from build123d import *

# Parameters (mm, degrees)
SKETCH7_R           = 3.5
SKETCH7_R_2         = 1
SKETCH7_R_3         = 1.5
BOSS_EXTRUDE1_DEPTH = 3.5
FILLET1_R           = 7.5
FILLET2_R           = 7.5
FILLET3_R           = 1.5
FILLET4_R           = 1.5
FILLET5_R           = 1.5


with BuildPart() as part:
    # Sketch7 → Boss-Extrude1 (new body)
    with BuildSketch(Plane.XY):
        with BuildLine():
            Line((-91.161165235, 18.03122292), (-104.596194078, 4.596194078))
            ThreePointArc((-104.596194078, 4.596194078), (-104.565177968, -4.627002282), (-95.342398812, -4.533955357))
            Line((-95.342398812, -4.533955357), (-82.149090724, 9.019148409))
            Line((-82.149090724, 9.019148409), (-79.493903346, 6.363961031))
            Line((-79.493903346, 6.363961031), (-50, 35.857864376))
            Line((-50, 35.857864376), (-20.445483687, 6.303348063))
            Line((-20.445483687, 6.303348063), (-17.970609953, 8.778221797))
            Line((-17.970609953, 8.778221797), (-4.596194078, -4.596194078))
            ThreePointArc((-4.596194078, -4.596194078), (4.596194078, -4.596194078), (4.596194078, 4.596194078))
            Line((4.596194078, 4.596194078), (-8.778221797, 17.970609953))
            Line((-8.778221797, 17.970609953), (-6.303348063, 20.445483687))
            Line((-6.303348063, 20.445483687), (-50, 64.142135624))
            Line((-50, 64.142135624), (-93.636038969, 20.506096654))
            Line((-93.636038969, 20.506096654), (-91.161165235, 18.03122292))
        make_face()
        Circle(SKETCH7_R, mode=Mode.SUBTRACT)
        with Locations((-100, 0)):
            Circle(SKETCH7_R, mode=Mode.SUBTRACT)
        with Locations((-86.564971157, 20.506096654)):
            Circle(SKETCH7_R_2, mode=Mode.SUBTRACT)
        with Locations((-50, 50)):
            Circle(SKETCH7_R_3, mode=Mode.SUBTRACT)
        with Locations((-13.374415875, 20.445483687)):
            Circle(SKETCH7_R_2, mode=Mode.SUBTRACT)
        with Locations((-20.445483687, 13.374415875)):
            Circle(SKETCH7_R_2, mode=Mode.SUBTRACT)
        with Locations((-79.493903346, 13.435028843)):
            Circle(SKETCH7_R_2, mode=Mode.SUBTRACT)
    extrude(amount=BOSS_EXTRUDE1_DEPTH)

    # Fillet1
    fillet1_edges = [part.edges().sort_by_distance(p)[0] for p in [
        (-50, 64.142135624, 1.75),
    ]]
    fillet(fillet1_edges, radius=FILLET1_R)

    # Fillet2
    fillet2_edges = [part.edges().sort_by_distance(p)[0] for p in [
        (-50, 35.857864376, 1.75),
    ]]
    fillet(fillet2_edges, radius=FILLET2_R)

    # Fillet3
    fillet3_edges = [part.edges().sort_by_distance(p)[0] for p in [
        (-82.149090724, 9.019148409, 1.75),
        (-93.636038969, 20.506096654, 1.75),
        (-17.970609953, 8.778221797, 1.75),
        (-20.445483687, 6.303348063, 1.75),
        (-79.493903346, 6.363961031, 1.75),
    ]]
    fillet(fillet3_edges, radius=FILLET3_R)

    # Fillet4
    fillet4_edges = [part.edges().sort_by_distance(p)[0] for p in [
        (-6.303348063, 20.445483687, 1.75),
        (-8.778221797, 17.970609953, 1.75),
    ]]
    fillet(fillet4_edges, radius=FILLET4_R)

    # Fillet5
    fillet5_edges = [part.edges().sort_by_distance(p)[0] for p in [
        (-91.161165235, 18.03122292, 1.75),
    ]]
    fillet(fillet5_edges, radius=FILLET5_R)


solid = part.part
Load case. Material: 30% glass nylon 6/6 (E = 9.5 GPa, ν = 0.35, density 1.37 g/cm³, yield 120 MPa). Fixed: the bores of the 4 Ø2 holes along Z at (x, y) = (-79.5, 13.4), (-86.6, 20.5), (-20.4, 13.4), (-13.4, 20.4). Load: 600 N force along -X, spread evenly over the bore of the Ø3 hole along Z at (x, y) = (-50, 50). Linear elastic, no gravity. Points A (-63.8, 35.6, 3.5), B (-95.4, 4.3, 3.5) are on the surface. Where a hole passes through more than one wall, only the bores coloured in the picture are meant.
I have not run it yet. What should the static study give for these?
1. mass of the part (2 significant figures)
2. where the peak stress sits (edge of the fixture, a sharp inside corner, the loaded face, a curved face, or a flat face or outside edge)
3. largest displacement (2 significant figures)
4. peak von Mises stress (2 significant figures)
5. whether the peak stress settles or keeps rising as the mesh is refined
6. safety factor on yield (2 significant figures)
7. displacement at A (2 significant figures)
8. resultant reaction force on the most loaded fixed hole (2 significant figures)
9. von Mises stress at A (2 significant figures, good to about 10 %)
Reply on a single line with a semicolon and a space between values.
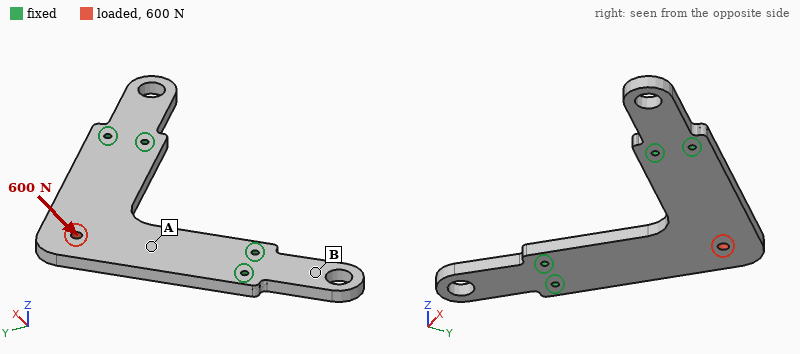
12 g; the loaded face; 53 µm; 32 MPa; settles; 3.7; 22 µm; 270 N; 5.5 MPa
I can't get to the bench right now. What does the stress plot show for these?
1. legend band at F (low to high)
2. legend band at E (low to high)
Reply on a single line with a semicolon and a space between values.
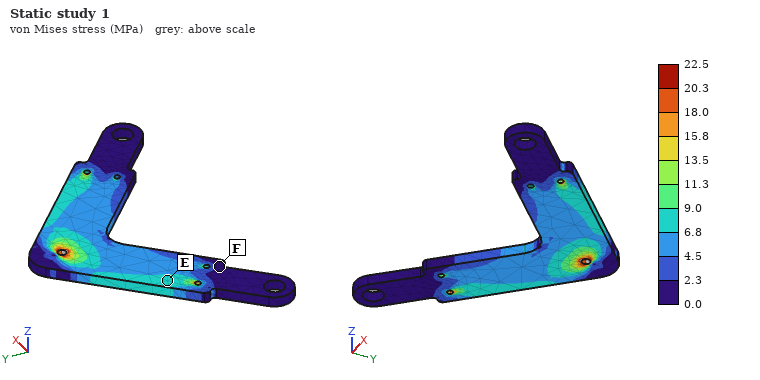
0.0 to 2.3 MPa; 6.8 to 9.0 MPa
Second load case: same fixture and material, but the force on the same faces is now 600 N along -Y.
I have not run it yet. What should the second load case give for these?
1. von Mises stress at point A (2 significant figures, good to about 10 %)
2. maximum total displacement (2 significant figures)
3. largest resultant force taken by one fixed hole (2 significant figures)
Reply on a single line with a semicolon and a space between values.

6.1 MPa; 47 µm; 270 N
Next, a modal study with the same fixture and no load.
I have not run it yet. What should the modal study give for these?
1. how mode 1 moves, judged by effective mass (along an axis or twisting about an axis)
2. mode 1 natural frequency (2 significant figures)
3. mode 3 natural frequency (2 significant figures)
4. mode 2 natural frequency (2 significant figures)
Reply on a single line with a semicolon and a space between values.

along Z; 800 Hz; 2100 Hz; 2100 Hz
